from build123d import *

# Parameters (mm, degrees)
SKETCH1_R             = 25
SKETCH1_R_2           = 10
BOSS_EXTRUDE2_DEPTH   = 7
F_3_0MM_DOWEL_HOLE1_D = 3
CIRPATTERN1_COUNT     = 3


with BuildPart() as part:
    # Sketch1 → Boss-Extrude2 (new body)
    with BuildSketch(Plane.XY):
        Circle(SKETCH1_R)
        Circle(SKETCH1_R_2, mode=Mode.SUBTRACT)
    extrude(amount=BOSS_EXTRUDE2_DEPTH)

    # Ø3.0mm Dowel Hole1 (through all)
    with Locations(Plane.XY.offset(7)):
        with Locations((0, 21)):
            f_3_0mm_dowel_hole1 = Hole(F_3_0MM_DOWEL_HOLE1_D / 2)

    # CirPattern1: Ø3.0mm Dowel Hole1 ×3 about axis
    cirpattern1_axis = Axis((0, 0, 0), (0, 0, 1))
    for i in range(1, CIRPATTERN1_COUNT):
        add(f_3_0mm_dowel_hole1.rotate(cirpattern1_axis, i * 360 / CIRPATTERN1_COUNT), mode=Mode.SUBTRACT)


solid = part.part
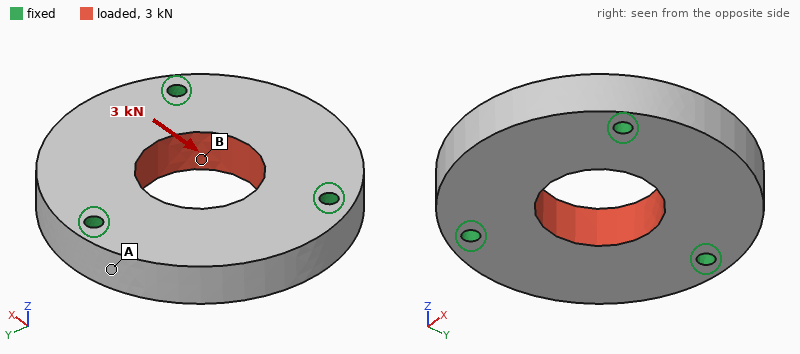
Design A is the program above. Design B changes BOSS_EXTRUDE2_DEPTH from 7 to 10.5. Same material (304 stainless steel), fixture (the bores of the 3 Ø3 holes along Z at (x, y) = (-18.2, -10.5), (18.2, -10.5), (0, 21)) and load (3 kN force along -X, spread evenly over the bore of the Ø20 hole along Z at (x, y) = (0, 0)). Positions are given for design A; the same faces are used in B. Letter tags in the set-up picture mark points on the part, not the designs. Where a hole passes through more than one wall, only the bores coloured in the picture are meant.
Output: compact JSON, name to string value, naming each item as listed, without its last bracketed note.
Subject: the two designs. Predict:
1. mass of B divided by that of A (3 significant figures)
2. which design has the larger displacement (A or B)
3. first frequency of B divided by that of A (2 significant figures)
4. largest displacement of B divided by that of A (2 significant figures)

{"mass of B divided by that of A": "1.50", "which design has the larger displacement": "A", "first frequency of B divided by that of A": "1.3", "largest displacement of B divided by that of A": "0.67"}
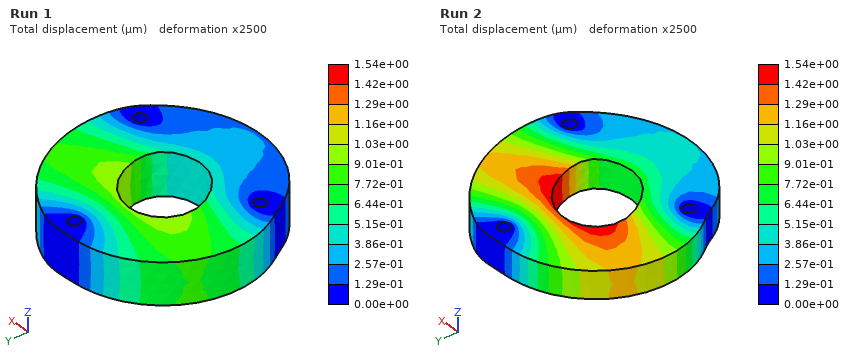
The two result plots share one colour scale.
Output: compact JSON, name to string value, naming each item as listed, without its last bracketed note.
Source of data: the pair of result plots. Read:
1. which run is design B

{"which run is design B": "Run 1"}
